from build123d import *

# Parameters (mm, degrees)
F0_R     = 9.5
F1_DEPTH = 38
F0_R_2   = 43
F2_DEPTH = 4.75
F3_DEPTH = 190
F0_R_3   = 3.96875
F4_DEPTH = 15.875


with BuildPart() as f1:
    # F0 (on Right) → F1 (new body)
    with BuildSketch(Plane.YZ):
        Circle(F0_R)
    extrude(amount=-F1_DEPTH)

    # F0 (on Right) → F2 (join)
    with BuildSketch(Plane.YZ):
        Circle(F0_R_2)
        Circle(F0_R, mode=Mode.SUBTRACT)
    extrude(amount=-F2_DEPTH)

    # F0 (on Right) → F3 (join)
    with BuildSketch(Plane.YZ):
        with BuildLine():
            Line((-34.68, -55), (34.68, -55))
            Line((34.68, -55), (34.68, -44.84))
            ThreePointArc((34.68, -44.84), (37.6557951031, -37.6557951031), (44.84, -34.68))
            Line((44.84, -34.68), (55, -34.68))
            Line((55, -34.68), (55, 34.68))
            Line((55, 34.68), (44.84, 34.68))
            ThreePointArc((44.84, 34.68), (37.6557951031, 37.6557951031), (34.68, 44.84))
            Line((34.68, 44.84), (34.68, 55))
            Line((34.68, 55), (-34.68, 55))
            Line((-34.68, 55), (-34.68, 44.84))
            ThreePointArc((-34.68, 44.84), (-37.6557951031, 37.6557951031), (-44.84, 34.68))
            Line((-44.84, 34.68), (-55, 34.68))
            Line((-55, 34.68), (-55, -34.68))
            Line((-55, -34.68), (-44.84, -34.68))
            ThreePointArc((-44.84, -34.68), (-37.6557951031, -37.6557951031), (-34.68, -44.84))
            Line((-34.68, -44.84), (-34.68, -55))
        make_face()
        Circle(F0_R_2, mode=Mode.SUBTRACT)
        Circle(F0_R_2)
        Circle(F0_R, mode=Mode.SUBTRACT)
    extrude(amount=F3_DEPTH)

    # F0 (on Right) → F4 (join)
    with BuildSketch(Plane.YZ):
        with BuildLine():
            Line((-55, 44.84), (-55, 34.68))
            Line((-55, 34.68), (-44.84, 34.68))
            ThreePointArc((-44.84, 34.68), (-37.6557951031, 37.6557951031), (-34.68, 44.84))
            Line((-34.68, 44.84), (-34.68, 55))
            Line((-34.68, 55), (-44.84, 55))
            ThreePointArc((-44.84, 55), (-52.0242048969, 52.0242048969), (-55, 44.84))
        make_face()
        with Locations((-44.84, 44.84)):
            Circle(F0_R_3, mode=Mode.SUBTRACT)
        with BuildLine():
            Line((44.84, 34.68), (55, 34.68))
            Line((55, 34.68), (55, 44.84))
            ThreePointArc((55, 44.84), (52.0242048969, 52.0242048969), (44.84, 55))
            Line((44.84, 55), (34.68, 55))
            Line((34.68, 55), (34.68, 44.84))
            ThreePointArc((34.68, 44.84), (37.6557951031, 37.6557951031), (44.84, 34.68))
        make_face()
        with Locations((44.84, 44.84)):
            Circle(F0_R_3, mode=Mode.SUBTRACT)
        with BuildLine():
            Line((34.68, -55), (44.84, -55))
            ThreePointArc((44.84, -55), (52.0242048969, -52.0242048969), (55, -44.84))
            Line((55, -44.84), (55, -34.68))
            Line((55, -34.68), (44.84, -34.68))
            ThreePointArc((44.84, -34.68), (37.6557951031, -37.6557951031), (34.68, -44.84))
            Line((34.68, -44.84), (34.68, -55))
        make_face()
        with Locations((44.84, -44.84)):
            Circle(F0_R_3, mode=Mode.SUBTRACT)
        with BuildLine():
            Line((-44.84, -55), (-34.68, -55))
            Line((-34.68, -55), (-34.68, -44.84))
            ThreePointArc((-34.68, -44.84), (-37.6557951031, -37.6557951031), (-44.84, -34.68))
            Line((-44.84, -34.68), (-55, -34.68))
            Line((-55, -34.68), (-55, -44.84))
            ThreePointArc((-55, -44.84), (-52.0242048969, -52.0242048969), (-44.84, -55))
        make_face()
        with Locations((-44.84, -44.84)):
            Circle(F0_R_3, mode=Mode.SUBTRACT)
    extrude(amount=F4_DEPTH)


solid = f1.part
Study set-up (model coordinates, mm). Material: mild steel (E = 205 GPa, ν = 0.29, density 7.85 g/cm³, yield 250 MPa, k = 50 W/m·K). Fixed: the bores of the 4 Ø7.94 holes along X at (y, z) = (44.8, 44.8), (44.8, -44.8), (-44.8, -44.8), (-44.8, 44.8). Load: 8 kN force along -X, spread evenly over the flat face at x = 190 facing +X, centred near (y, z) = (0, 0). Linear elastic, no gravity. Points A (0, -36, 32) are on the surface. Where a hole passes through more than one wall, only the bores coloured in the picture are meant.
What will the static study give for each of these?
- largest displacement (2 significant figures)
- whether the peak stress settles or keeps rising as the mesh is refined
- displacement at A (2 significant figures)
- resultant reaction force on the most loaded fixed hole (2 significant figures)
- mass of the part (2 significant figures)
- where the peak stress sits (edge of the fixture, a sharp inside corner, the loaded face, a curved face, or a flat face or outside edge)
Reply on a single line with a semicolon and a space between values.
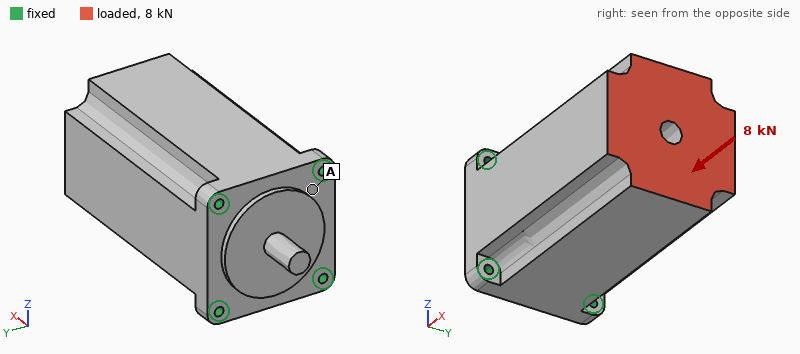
1.7 µm; keeps rising; 0.84 µm; 2.1 kN; 16 kg; edge of the fixture
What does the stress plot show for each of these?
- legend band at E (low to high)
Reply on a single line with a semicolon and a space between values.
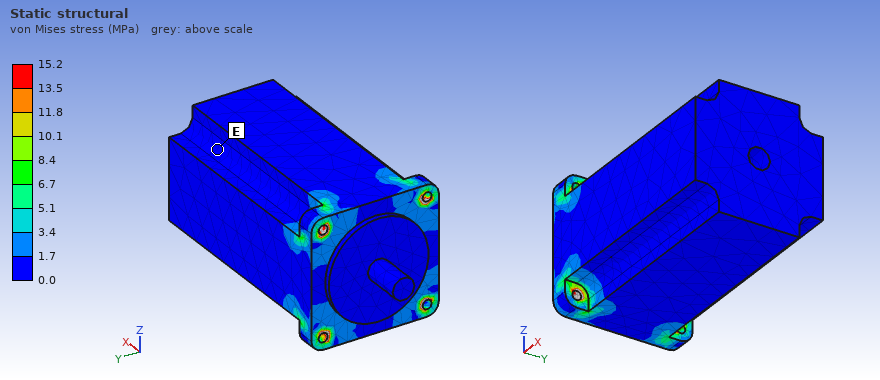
0.0 to 1.7 MPa
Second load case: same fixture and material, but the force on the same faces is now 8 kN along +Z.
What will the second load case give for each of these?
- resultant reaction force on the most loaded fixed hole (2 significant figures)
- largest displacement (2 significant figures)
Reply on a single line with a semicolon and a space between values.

8.9 kN; 29 µm
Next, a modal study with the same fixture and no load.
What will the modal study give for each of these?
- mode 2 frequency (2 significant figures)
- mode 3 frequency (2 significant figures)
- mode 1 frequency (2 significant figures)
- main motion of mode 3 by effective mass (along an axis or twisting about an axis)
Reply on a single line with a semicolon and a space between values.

1200 Hz; 3300 Hz; 1200 Hz; along X
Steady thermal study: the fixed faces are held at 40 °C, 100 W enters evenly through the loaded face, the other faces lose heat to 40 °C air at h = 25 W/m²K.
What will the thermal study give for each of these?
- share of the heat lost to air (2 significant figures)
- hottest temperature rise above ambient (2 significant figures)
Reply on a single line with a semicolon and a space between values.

46 %; 34 K
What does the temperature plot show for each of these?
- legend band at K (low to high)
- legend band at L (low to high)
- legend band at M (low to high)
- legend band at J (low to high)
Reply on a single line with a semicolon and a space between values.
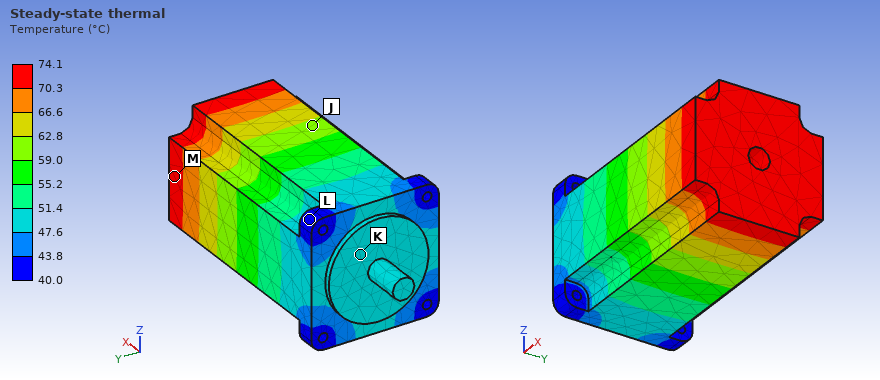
47.6 to 51.4 °C; 40.0 to 43.8 °C; 70.3 to 74.1 °C; 59.0 to 62.8 °C
